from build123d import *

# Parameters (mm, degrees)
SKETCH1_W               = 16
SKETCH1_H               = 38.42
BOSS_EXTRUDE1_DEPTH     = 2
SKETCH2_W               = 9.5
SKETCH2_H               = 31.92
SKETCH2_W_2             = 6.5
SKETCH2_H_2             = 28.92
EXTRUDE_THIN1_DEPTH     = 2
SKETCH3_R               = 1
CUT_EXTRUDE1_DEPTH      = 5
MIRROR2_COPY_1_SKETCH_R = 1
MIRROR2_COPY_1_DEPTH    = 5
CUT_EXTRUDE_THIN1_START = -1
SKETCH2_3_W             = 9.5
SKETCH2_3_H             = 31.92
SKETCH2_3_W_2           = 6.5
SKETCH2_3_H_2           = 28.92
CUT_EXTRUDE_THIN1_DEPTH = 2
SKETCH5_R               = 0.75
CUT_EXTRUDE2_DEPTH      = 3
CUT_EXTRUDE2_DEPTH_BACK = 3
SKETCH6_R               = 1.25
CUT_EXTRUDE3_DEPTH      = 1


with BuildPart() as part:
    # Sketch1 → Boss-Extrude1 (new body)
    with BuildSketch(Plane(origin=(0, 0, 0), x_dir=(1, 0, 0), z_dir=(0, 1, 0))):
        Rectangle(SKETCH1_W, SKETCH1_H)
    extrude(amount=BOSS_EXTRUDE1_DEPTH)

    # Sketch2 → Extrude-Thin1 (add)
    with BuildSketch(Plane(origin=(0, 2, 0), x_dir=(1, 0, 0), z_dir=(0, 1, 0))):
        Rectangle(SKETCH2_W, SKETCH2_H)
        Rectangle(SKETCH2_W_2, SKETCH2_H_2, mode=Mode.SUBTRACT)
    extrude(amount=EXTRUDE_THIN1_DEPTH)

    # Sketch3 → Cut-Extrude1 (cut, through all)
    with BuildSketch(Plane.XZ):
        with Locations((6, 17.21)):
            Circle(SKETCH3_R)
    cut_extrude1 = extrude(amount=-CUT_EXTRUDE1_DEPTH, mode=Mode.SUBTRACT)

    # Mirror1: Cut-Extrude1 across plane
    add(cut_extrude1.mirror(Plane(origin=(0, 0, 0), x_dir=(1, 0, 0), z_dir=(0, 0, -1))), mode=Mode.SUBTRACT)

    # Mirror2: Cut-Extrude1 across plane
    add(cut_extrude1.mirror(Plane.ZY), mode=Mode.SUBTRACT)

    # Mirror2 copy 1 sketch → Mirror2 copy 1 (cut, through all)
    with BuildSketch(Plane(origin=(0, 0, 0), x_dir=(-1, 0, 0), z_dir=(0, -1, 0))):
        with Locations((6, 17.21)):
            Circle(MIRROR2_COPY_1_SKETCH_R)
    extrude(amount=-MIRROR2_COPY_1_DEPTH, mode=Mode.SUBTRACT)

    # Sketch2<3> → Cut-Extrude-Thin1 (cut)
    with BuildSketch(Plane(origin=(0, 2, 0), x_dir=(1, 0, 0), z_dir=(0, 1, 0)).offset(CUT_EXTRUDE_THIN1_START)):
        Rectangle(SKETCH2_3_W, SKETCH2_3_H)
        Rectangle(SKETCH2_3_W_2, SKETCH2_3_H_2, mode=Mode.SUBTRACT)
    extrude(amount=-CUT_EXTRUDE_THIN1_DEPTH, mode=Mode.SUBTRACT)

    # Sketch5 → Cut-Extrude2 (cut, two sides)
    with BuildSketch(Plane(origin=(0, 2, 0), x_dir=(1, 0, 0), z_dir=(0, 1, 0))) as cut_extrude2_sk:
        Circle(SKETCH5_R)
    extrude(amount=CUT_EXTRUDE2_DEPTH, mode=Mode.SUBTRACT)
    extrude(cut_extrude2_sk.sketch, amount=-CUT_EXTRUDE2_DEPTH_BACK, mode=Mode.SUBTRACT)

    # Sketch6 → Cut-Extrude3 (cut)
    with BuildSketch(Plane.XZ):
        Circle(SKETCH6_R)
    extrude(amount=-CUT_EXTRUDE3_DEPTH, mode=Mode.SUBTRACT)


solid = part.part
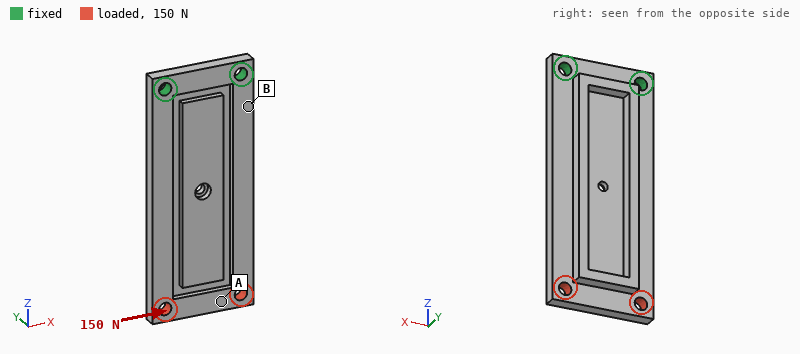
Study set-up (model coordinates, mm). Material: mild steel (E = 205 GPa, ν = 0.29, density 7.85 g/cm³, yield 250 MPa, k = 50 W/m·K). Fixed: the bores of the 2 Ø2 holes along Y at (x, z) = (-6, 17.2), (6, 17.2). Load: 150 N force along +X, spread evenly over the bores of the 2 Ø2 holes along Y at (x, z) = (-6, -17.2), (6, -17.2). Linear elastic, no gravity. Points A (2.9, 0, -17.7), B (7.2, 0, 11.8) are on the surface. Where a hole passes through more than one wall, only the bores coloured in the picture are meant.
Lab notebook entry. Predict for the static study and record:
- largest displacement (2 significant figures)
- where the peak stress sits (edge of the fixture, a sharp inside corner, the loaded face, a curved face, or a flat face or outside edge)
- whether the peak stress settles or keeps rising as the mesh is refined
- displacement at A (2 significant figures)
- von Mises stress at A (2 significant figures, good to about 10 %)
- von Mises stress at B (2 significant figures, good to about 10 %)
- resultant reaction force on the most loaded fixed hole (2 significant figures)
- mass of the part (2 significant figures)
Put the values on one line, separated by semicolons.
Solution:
21 µm; edge of the fixture; keeps rising; 19 µm; 10 MPa; 47 MPa; 420 N; 10 g
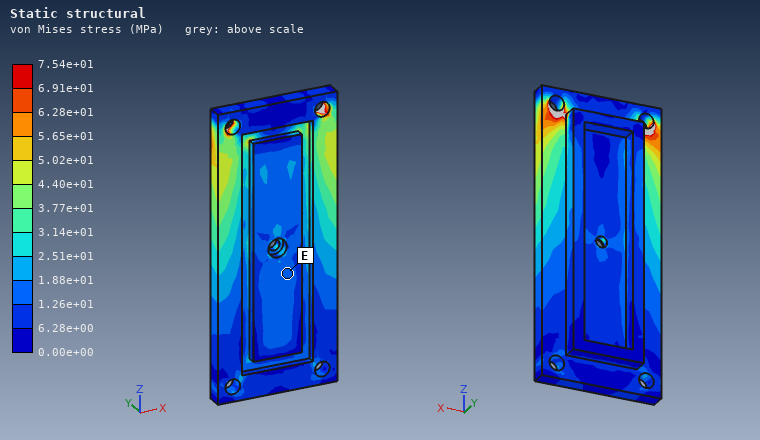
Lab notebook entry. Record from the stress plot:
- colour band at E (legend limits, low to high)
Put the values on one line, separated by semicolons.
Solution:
1.26e+01 to 1.88e+01 MPa
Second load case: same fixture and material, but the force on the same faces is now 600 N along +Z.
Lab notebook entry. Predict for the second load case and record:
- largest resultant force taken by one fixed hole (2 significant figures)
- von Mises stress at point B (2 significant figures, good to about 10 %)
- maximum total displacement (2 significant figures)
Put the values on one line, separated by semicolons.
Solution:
300 N; 38 MPa; 30 µm
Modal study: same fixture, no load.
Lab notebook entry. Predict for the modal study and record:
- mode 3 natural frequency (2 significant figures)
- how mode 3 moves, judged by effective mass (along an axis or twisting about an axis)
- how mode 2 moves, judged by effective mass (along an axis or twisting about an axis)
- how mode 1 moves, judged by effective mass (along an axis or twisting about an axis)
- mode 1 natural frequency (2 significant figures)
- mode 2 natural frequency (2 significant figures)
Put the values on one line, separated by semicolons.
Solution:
8400 Hz; along X; twisting about Z; along Y; 1500 Hz; 5500 Hz
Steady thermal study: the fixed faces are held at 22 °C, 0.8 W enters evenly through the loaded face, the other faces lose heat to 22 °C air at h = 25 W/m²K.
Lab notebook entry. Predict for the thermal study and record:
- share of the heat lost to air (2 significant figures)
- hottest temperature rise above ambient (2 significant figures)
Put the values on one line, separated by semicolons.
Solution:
36 %; 14 K
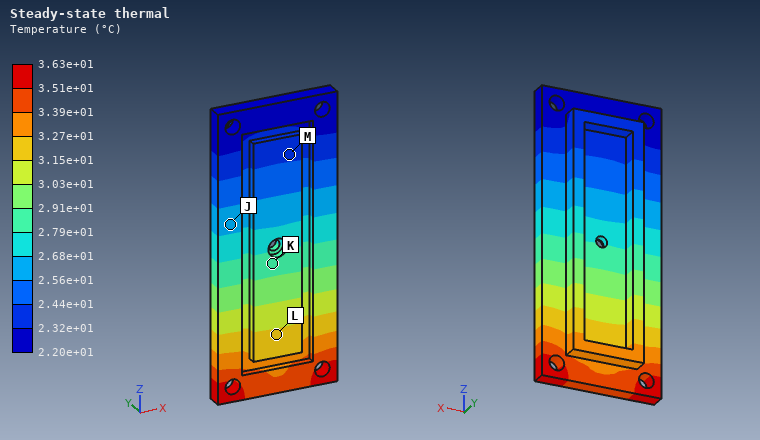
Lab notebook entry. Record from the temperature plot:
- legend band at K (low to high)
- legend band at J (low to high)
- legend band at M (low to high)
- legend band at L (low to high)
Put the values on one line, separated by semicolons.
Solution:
2.79e+01 to 2.91e+01 °C; 2.56e+01 to 2.68e+01 °C; 2.32e+01 to 2.44e+01 °C; 3.15e+01 to 3.27e+01 °C
